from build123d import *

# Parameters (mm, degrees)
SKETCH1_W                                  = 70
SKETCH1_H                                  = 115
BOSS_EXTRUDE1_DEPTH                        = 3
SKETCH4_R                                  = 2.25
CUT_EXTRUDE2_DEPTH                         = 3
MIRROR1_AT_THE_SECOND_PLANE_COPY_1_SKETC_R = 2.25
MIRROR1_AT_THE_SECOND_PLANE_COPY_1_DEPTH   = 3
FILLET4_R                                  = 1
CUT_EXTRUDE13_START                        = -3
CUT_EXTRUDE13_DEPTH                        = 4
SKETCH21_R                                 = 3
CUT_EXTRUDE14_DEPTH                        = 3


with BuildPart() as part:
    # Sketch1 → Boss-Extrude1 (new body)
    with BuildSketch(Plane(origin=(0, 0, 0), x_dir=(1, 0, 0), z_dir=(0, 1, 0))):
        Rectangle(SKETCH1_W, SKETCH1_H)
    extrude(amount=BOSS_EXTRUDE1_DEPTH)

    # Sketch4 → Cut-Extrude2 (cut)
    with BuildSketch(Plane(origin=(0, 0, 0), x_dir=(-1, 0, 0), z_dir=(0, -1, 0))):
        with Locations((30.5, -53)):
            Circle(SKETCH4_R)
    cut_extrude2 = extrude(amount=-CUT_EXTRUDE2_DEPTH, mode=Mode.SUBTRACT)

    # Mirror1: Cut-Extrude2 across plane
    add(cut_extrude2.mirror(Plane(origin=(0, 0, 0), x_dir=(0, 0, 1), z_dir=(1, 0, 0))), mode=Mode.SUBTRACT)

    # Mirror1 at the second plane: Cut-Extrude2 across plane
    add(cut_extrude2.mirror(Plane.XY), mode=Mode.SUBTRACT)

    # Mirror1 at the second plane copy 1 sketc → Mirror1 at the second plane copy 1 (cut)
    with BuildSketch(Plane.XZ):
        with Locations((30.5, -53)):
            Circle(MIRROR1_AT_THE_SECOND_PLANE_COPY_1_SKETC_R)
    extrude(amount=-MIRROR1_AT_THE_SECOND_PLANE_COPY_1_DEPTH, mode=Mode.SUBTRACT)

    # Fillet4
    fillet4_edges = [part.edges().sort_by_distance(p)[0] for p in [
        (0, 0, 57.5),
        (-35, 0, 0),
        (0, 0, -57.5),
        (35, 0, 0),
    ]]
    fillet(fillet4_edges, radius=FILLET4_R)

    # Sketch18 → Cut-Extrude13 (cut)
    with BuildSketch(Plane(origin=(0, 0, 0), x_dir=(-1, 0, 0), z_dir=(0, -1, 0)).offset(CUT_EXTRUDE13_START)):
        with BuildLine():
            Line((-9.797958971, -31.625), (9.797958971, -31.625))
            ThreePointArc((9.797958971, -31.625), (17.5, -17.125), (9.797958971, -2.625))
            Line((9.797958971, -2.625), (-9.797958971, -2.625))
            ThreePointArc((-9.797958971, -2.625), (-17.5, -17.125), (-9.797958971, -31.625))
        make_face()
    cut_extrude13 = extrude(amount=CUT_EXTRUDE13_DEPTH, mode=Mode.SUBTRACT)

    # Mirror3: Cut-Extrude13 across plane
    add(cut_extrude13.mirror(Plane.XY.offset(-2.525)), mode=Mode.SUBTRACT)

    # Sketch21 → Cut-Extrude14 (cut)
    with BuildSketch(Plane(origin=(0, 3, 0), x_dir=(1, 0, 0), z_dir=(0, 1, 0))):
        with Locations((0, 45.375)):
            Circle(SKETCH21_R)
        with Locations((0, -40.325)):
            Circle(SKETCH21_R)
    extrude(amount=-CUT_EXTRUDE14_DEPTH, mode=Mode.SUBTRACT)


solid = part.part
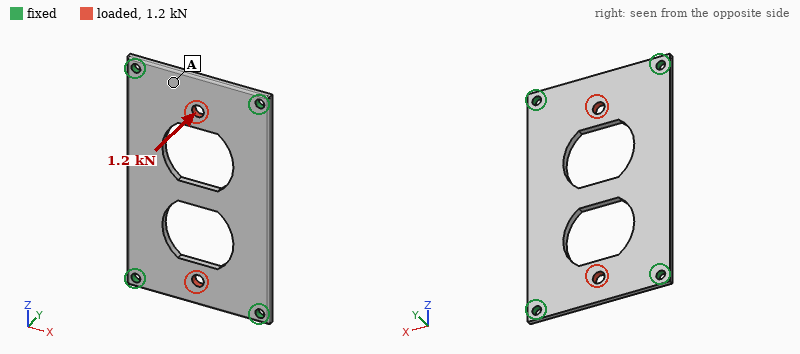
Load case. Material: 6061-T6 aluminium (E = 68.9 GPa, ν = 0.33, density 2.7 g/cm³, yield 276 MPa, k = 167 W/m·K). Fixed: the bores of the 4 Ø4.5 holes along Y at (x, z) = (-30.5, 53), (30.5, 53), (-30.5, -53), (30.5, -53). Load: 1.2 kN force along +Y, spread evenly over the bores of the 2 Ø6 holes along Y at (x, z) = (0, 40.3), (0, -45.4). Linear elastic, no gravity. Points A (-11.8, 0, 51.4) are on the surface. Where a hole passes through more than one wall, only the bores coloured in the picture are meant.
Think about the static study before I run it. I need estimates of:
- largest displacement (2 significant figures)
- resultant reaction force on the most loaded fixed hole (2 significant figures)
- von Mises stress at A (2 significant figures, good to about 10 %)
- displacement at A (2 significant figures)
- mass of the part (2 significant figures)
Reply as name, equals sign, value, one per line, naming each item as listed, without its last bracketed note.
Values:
largest displacement = 0.38 mm
resultant reaction force on the most loaded fixed hole = 310 N
von Mises stress at A = 41 MPa
displacement at A = 0.13 mm
mass of the part = 50 g
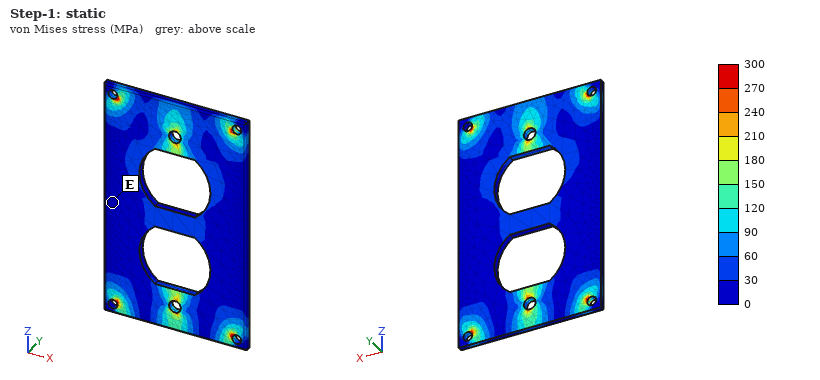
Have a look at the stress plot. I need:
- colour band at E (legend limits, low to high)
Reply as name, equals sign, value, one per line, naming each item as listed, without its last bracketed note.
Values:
colour band at E = 0 to 30 MPa
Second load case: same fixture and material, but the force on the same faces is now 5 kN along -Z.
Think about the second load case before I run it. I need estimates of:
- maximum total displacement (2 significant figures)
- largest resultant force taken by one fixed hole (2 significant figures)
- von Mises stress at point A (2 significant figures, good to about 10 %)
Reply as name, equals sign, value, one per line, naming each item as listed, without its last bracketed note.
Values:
maximum total displacement = 43 µm
largest resultant force taken by one fixed hole = 1.5 kN
von Mises stress at point A = 25 MPa
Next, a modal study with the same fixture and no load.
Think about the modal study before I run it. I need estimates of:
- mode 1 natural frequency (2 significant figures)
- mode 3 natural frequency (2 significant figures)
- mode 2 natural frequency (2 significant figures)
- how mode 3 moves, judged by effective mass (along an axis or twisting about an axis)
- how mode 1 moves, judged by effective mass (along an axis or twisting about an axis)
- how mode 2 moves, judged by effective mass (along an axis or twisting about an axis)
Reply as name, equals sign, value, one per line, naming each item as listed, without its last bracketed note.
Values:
mode 1 natural frequency = 1300 Hz
mode 3 natural frequency = 3200 Hz
mode 2 natural frequency = 1800 Hz
how mode 3 moves, judged by effective mass = twisting about X
how mode 1 moves, judged by effective mass = along Y
how mode 2 moves, judged by effective mass = twisting about Z
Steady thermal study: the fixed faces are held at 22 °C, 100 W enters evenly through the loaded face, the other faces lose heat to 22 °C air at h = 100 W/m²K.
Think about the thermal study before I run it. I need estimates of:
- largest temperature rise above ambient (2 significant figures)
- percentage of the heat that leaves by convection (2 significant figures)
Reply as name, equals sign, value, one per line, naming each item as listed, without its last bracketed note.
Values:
largest temperature rise above ambient = 69 K
percentage of the heat that leaves by convection = 31 %
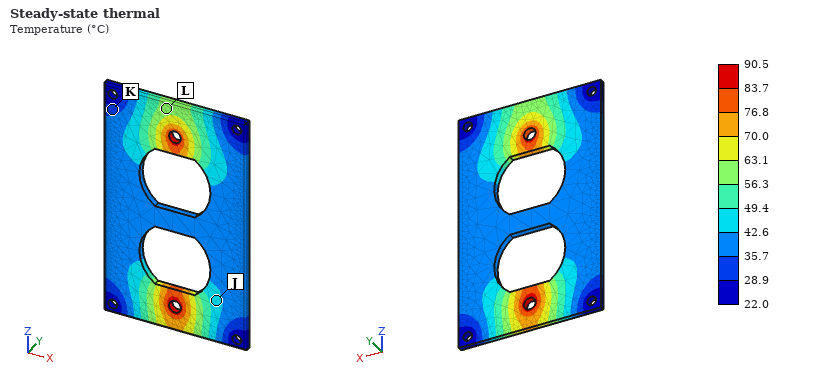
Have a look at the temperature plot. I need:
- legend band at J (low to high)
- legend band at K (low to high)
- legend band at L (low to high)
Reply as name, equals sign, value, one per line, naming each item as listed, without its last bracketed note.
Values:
legend band at J = 42.6 to 49.4 °C
legend band at K = 28.9 to 35.7 °C
legend band at L = 56.3 to 63.1 °C
